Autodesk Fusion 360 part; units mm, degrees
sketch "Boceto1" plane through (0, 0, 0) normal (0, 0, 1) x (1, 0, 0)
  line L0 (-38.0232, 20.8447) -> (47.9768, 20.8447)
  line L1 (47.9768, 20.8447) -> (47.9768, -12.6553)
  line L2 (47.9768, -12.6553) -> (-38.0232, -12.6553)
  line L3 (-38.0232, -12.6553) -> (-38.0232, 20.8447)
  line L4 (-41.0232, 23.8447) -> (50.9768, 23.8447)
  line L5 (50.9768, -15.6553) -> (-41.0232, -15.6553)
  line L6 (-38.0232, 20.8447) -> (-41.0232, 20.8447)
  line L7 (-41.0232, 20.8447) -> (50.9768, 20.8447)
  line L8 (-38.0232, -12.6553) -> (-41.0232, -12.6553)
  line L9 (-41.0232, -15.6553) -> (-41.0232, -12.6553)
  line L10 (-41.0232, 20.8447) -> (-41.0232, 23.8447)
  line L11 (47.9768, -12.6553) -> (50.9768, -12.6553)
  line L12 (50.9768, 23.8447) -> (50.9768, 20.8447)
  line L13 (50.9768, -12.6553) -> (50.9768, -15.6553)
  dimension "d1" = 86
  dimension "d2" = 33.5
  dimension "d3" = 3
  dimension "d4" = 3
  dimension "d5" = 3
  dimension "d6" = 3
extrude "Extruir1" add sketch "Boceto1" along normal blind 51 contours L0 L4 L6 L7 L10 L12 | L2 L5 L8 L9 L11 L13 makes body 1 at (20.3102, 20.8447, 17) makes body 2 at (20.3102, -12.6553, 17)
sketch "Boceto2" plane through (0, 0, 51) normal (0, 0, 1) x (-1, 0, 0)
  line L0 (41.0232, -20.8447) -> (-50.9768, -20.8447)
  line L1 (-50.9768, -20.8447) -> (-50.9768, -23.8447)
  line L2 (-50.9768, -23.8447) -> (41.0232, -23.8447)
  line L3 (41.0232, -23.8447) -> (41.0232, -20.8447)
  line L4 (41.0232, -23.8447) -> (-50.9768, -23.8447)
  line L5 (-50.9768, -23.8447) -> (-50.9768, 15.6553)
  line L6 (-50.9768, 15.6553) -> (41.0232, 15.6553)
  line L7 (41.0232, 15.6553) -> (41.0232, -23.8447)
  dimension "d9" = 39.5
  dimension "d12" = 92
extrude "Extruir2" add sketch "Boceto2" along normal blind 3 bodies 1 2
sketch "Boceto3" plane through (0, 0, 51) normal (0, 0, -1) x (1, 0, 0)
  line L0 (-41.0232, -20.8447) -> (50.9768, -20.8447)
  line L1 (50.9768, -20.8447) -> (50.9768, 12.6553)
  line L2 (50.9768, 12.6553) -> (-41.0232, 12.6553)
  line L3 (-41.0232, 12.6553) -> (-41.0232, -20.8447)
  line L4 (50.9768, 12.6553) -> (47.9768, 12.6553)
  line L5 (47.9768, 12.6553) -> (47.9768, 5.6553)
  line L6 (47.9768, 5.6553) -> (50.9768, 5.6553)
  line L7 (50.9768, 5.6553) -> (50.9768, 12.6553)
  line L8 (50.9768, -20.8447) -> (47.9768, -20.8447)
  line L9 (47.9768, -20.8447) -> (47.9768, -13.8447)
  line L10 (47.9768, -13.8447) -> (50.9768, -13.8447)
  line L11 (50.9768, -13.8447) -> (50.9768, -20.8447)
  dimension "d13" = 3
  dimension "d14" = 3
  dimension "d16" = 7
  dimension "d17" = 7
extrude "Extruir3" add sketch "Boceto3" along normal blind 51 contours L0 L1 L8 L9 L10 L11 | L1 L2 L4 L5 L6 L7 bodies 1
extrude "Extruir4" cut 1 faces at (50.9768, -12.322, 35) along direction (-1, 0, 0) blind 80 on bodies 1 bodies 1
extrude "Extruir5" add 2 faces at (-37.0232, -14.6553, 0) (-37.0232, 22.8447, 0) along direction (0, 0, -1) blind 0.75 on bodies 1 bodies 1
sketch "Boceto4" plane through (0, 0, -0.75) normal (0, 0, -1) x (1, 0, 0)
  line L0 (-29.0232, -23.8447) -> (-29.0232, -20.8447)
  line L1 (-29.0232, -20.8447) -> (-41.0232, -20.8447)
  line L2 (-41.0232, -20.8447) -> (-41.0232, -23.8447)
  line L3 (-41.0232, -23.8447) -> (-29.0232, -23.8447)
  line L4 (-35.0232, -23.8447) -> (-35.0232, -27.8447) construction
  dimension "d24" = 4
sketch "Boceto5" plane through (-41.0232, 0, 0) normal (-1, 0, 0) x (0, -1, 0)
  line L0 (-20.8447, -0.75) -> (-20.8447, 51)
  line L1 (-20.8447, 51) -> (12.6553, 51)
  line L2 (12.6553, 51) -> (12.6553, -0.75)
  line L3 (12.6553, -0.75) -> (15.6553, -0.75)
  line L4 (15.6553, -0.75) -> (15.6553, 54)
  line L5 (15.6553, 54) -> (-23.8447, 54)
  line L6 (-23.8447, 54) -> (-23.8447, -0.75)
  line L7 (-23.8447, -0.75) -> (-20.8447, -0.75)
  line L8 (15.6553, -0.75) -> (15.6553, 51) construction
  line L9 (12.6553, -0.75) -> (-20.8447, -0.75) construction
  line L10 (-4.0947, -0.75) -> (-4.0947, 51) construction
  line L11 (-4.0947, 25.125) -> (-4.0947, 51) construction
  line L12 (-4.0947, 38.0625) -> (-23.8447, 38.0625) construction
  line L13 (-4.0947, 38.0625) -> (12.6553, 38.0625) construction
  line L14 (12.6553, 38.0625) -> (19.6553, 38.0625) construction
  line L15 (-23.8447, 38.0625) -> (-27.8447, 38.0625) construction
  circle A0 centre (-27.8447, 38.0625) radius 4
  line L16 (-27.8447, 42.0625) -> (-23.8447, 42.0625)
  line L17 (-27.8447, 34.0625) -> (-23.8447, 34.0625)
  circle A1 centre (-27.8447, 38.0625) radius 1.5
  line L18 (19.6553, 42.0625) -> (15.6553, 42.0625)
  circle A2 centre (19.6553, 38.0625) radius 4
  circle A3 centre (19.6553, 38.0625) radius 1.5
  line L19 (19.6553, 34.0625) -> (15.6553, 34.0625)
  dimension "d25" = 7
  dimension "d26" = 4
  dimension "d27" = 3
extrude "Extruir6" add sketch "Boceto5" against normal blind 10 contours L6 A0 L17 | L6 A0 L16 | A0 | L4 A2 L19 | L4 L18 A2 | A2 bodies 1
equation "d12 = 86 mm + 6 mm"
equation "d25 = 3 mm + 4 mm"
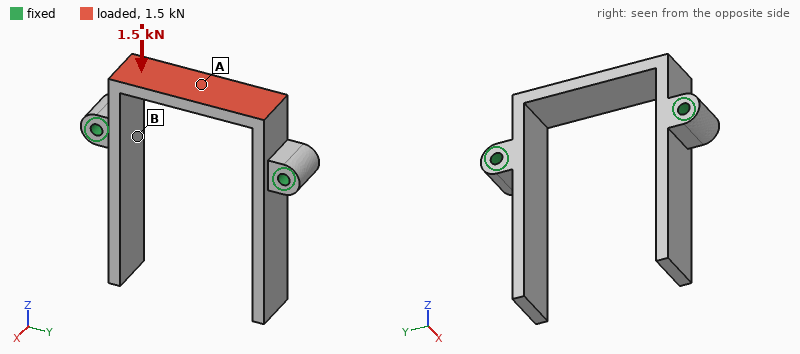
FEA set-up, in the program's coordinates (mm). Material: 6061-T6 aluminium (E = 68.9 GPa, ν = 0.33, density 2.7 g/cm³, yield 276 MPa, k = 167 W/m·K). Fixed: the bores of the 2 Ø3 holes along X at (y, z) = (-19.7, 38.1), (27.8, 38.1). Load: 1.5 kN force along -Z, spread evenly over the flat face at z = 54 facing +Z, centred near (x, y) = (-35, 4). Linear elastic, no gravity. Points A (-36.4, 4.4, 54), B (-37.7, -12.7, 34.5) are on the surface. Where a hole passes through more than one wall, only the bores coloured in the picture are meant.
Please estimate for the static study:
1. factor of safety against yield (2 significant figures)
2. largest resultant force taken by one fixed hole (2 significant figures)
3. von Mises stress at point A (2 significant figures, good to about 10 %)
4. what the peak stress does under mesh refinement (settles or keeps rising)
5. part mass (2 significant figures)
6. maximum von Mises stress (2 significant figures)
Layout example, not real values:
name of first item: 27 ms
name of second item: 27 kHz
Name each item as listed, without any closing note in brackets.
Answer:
factor of safety against yield: 1.7
largest resultant force taken by one fixed hole: 880 N
von Mises stress at point A: 140 MPa
what the peak stress does under mesh refinement: settles
part mass: 17 g
maximum von Mises stress: 160 MPa
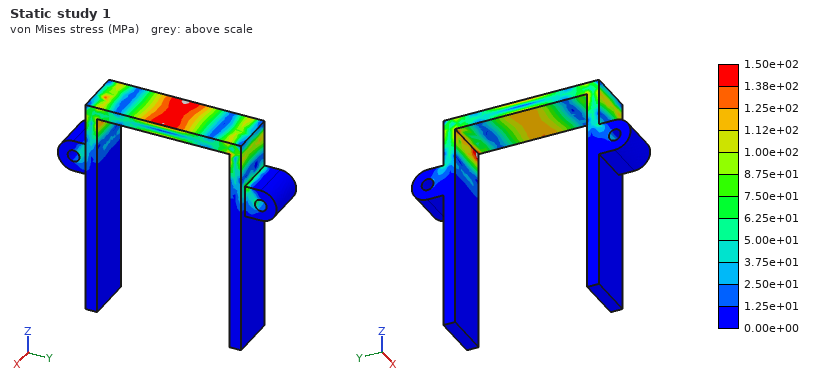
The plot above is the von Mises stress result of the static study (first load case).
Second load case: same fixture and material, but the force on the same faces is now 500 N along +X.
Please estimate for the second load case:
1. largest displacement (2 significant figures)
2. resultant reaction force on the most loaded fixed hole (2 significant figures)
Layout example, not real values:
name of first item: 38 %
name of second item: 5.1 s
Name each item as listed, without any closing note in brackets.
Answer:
largest displacement: 39 µm
resultant reaction force on the most loaded fixed hole: 250 N
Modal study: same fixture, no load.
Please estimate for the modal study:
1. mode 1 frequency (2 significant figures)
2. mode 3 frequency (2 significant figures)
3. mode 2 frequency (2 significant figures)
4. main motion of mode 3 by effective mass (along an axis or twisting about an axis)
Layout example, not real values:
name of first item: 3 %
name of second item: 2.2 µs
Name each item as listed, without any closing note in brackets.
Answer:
mode 1 frequency: 1800 Hz
mode 3 frequency: 5100 Hz
mode 2 frequency: 1800 Hz
main motion of mode 3 by effective mass: along X
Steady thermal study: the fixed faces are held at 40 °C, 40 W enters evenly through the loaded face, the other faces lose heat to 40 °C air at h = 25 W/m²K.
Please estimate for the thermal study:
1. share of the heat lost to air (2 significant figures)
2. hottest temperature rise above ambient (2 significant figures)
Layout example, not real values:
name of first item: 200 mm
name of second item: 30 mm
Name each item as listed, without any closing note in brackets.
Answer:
share of the heat lost to air: 4.2 %
hottest temperature rise above ambient: 70 K
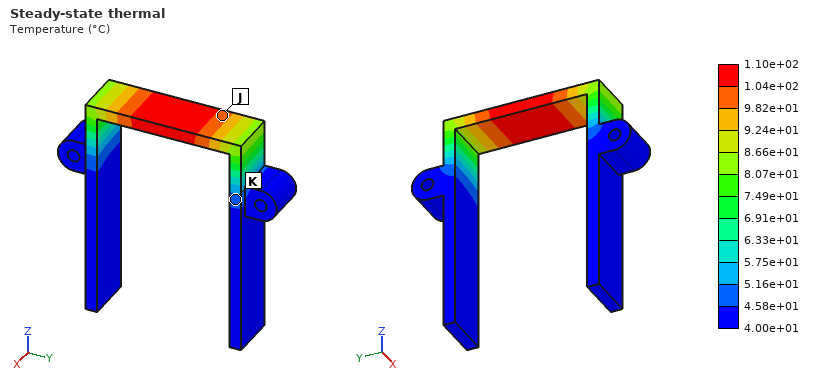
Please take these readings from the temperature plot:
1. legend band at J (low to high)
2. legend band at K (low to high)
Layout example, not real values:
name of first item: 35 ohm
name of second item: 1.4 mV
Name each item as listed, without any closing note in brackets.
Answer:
legend band at J: 9.82e+01 to 1.04e+02 °C
legend band at K: 4.58e+01 to 5.16e+01 °C
